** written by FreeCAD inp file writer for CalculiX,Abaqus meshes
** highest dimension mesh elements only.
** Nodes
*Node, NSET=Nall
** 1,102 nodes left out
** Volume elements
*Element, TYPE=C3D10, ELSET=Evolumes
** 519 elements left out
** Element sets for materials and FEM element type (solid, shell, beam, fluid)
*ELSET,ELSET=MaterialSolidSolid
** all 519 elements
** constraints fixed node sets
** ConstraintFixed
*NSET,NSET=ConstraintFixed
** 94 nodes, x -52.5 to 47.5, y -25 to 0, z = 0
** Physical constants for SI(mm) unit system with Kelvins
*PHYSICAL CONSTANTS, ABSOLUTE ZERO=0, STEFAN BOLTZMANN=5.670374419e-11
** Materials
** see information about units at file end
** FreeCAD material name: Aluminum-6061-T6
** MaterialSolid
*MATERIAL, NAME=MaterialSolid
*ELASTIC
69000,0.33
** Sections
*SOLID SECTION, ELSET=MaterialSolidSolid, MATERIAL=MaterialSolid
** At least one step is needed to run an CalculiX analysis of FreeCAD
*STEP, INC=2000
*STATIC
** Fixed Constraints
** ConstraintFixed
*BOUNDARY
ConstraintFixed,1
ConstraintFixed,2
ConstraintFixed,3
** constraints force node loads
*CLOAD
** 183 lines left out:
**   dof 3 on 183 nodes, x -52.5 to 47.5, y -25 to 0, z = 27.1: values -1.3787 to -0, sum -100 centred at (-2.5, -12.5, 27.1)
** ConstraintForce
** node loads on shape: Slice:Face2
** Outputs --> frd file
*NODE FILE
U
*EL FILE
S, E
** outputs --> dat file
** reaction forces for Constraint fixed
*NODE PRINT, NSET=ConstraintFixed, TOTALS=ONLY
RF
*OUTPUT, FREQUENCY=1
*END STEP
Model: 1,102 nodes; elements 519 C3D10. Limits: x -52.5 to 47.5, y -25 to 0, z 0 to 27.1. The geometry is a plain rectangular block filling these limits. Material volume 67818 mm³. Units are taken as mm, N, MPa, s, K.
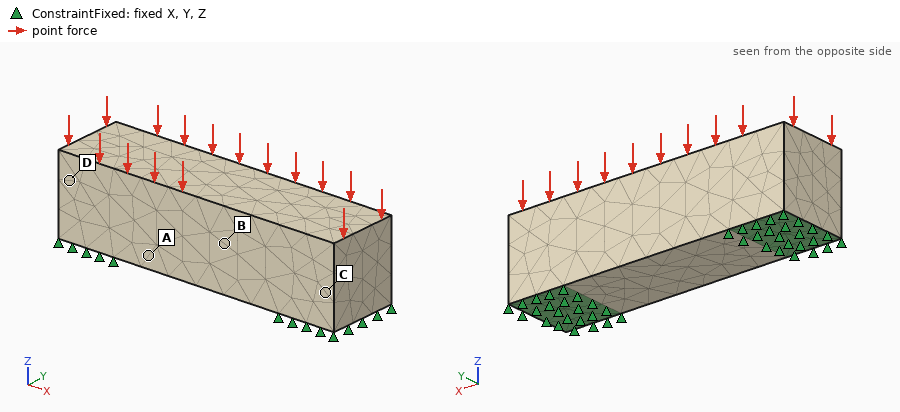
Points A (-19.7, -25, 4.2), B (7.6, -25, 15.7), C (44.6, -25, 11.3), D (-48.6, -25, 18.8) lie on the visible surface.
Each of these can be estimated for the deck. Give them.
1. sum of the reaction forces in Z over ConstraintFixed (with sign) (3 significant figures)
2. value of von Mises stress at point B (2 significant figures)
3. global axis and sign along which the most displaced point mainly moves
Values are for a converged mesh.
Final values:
100 N
0.056 MPa
-Z
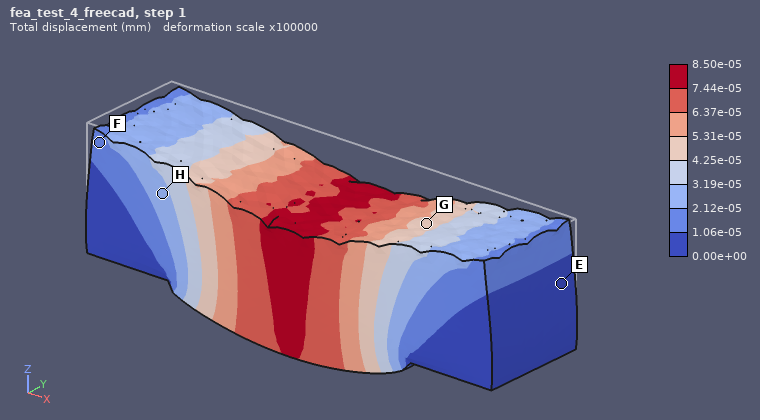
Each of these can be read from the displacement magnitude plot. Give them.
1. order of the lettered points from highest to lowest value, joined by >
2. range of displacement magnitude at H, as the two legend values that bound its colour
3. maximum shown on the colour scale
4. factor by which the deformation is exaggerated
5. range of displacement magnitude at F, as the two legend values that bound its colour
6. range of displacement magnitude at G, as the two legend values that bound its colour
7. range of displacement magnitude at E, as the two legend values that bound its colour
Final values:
G > H > F > E
2.12e-05 to 3.19e-05 mm
8.50e-05 mm
100000
1.06e-05 to 2.12e-05 mm
4.25e-05 to 5.31e-05 mm
0.00e+00 to 1.06e-05 mm
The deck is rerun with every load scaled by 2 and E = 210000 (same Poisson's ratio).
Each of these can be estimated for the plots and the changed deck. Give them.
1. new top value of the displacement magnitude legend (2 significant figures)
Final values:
5.6e-05 mm
